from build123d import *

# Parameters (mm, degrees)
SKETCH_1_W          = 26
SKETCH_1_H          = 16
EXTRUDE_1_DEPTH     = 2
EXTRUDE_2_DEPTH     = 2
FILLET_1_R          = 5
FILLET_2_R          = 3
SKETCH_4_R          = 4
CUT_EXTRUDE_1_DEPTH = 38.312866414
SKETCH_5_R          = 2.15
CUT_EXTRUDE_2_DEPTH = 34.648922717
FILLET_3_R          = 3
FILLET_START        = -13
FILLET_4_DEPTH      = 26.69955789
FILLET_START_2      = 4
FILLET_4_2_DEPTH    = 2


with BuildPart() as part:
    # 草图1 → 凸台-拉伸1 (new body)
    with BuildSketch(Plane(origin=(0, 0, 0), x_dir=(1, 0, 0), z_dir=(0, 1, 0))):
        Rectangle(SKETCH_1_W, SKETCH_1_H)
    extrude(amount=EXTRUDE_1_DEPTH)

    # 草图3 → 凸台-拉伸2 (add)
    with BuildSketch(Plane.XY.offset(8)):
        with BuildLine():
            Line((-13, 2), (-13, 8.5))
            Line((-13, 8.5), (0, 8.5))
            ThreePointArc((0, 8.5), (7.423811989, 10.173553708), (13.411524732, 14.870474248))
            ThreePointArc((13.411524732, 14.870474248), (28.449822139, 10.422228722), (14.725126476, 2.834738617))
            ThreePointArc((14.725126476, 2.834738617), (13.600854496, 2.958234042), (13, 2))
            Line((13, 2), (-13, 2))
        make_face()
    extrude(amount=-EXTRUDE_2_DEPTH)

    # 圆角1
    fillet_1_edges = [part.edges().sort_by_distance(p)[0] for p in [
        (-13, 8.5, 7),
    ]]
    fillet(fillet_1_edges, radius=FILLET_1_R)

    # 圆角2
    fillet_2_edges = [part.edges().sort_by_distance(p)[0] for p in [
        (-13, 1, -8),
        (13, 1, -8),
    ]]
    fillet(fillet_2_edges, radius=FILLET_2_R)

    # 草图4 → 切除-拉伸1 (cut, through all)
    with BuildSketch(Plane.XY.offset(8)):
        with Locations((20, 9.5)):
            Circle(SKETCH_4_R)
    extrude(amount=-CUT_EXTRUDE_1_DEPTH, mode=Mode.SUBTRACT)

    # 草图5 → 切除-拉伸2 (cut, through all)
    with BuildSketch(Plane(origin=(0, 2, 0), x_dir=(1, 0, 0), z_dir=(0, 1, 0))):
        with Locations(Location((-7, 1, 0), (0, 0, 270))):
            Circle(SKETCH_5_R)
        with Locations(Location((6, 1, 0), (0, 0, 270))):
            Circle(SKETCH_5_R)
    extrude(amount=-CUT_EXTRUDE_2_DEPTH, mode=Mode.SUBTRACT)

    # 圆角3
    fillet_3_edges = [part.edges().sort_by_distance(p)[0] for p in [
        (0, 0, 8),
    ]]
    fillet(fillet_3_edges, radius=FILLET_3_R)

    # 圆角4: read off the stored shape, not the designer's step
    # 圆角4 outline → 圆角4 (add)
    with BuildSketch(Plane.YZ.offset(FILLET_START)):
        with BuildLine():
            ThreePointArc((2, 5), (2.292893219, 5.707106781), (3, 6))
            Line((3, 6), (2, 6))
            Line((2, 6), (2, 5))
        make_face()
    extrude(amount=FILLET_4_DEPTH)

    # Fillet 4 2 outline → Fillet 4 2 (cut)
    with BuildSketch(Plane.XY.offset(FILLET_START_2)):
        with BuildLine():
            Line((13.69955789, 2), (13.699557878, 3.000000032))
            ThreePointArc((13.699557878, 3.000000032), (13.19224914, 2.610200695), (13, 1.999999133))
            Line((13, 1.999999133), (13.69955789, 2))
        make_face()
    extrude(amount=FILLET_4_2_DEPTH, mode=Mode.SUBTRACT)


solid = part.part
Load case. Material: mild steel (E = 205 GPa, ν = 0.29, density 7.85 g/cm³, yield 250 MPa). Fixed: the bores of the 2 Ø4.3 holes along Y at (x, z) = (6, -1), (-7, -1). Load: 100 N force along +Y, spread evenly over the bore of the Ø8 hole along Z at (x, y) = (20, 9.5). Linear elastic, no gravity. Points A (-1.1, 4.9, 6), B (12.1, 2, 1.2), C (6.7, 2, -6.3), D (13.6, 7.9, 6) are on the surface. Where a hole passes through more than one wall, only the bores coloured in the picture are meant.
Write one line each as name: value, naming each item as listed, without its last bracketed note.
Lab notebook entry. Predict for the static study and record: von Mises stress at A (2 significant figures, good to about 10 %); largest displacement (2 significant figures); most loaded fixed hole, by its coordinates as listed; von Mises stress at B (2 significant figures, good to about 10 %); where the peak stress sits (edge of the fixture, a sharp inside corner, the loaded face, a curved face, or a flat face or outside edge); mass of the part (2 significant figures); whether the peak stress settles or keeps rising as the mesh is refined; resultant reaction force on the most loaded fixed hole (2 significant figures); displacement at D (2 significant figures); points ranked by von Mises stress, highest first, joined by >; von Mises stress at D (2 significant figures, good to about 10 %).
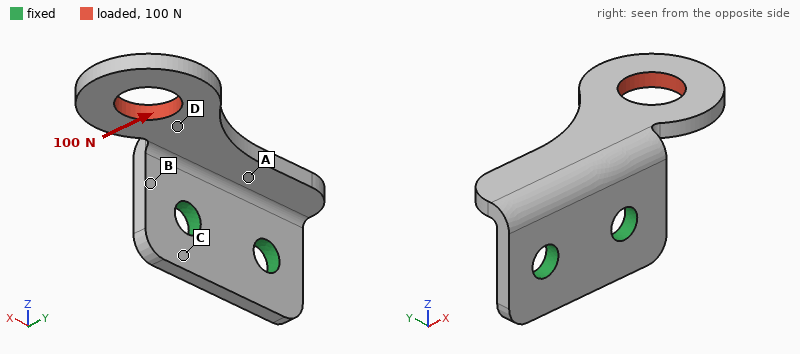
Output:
von Mises stress at A: 37 MPa
largest displacement: 46 µm
most loaded fixed hole, by its coordinates as listed: (6, -1)
von Mises stress at B: 65 MPa
where the peak stress sits: edge of the fixture
mass of the part: 11 g
whether the peak stress settles or keeps rising as the mesh is refined: keeps rising
resultant reaction force on the most loaded fixed hole: 170 N
displacement at D: 19 µm
points ranked by von Mises stress, highest first, joined by >: B > A > D > C
von Mises stress at D: 22 MPa
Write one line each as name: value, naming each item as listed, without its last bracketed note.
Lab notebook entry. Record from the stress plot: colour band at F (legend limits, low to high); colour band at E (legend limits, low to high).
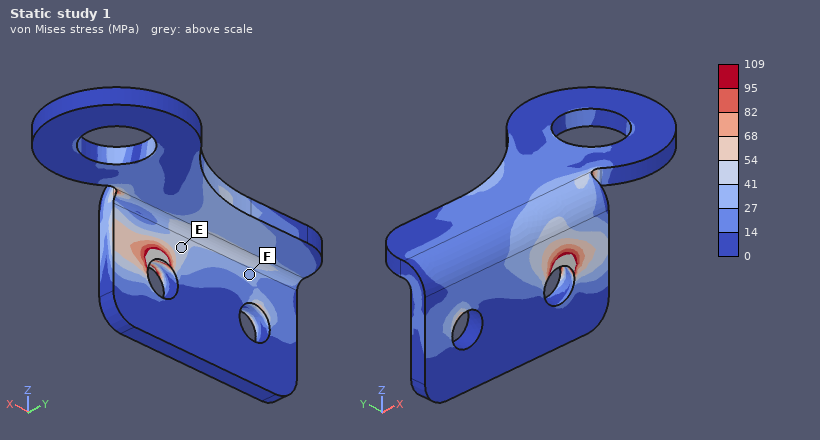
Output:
colour band at F: 27 to 41 MPa
colour band at E: 41 to 54 MPa
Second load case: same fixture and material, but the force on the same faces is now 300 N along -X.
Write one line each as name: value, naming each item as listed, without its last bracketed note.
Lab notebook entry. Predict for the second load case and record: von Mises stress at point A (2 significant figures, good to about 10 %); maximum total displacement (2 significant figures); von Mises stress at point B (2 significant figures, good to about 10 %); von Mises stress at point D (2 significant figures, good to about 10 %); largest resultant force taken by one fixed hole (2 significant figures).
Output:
von Mises stress at point A: 52 MPa
maximum total displacement: 44 µm
von Mises stress at point B: 51 MPa
von Mises stress at point D: 21 MPa
largest resultant force taken by one fixed hole: 260 N
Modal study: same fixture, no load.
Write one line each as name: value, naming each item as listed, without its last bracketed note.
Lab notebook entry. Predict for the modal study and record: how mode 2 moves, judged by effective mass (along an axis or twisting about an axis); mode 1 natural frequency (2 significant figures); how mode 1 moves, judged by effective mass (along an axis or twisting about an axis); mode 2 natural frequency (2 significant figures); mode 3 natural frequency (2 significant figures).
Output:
how mode 2 moves, judged by effective mass: along Y
mode 1 natural frequency: 2800 Hz
how mode 1 moves, judged by effective mass: along Z
mode 2 natural frequency: 5700 Hz
mode 3 natural frequency: 7100 Hz
